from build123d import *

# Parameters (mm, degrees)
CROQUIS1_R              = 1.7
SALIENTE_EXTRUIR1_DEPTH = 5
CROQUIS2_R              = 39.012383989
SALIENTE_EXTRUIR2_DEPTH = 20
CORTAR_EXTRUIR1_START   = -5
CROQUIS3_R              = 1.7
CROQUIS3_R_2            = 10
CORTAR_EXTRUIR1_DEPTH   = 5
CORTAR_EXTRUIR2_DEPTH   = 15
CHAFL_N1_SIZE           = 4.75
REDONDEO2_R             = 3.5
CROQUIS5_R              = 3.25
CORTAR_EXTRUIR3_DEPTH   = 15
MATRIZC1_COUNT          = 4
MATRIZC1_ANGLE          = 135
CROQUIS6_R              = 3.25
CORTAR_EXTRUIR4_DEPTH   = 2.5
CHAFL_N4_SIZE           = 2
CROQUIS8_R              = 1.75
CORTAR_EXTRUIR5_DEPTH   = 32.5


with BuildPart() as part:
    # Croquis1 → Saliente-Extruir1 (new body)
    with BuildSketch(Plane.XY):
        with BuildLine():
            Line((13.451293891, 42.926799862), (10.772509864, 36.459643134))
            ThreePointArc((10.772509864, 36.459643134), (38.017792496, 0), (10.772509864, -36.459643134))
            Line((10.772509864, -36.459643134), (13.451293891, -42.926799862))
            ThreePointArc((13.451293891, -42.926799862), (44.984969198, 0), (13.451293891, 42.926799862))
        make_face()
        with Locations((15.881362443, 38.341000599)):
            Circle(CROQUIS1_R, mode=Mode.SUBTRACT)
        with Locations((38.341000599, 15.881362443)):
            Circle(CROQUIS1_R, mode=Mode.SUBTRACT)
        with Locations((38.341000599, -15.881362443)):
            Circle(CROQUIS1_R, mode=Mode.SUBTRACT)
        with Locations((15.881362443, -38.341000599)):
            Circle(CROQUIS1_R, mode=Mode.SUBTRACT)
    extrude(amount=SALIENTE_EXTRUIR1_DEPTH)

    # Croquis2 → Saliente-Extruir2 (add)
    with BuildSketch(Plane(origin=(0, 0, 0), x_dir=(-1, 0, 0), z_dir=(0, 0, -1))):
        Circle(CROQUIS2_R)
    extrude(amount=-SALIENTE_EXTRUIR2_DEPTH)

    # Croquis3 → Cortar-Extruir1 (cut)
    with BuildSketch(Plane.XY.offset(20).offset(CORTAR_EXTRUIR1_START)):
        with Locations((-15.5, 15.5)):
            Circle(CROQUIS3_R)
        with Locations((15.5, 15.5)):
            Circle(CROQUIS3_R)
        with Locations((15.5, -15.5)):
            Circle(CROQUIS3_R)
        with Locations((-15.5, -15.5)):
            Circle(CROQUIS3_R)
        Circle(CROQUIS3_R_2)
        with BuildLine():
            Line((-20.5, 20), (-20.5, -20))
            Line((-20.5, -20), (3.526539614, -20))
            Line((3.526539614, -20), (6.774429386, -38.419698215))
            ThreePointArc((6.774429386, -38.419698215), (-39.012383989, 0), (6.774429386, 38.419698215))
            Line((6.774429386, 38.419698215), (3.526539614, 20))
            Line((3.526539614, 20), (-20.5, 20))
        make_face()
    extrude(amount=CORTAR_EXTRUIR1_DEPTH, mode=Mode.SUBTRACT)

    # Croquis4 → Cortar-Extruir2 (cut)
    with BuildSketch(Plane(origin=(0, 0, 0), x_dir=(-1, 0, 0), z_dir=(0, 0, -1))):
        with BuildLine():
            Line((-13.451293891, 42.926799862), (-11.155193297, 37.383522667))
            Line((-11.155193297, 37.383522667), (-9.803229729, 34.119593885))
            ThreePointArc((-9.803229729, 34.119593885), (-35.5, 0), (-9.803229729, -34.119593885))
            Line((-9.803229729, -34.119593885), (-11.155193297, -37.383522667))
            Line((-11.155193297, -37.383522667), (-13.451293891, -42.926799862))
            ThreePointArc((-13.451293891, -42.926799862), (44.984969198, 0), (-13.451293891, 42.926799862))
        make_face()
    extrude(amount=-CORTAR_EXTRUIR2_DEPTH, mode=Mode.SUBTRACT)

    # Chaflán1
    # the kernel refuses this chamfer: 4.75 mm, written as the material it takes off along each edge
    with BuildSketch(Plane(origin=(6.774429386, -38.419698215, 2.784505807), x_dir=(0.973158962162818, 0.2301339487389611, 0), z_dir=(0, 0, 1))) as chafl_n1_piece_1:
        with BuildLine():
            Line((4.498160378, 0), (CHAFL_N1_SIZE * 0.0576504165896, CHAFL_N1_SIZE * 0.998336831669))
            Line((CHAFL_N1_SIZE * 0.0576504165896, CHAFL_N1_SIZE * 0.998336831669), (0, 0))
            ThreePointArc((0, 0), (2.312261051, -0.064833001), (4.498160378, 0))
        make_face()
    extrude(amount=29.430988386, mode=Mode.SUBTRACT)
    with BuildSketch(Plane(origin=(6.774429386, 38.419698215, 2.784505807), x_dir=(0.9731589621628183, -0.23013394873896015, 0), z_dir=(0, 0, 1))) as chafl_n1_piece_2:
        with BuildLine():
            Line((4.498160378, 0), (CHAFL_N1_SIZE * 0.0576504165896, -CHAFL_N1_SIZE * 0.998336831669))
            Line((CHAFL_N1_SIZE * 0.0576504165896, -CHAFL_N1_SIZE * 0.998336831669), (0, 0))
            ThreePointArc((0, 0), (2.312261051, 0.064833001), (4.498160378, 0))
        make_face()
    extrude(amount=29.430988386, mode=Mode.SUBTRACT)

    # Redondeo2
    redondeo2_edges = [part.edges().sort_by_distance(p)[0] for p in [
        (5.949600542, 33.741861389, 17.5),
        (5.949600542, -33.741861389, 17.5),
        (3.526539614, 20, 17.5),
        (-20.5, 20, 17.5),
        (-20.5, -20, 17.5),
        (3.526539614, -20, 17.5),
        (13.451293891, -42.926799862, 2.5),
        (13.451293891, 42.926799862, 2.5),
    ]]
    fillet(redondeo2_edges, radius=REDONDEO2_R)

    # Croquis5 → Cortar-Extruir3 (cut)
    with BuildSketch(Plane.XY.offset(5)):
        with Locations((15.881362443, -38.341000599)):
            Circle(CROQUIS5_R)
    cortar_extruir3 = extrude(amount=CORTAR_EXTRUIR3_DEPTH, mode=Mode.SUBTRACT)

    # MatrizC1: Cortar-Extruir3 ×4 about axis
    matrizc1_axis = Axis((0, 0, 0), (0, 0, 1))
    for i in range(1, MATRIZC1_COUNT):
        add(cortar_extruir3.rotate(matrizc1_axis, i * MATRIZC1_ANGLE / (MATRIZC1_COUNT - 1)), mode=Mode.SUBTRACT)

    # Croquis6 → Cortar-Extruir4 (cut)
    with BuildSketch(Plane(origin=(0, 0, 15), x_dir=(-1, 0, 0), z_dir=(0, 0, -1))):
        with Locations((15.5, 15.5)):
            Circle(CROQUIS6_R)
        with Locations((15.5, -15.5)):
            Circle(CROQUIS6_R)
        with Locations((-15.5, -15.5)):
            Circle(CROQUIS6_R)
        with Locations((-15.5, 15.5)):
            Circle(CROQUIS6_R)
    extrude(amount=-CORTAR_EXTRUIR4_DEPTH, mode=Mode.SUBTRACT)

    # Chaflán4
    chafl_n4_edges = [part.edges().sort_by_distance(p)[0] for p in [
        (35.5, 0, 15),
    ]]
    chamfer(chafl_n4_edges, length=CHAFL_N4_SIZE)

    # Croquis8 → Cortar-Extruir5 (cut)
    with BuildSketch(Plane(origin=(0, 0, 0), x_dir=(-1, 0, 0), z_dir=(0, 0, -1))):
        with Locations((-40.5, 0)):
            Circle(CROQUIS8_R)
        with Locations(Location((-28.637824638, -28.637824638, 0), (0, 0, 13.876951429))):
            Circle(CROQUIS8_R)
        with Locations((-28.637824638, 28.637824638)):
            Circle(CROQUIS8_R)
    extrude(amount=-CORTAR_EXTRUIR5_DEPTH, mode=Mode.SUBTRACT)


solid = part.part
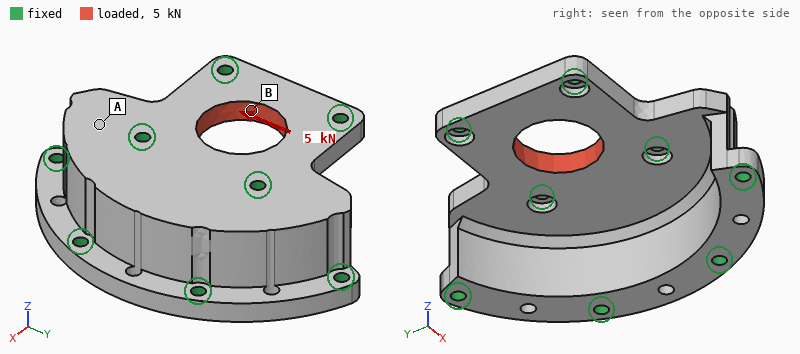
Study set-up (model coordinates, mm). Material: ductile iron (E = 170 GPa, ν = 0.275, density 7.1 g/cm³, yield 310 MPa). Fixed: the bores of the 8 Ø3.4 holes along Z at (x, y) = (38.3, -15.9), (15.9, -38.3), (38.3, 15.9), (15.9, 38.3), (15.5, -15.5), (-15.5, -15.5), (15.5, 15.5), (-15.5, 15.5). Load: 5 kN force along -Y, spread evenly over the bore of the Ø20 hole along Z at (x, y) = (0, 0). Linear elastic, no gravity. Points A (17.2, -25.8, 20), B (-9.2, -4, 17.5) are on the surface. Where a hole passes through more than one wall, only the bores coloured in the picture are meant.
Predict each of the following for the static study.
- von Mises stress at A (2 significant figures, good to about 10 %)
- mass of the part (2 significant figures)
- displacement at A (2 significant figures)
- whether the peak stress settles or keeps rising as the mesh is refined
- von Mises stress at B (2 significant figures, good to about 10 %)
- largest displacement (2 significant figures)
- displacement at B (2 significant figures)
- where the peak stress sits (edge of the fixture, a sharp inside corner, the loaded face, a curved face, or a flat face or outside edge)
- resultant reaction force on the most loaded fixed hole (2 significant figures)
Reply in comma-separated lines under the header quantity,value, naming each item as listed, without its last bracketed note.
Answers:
quantity,value
von Mises stress at A,9.3 MPa
mass of the part,150 g
displacement at A,1.4 µm
whether the peak stress settles or keeps rising as the mesh is refined,keeps rising
von Mises stress at B,31 MPa
largest displacement,4.1 µm
displacement at B,2.6 µm
where the peak stress sits,edge of the fixture
resultant reaction force on the most loaded fixed hole,1.4 kN
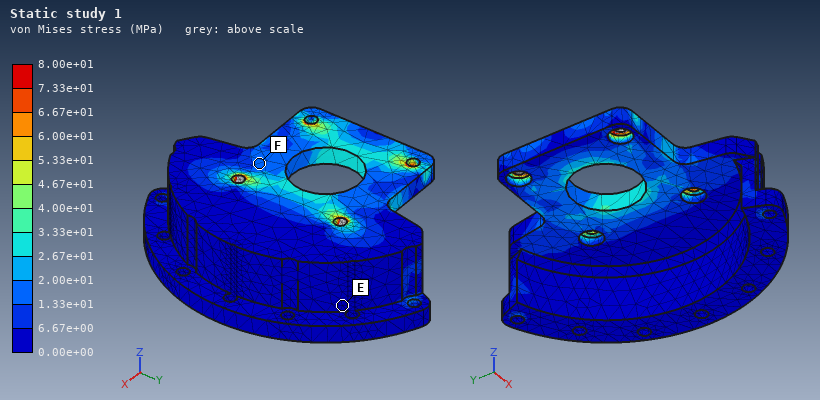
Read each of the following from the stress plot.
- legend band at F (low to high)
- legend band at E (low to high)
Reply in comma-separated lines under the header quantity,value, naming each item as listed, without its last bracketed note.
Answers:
quantity,value
legend band at F,1.33e+01 to 2.00e+01 MPa
legend band at E,0.00e+00 to 6.67e+00 MPa
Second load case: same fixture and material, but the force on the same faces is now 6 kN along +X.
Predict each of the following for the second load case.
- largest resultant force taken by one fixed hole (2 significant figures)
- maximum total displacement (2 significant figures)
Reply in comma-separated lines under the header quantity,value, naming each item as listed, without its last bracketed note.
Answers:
quantity,value
largest resultant force taken by one fixed hole,1.6 kN
maximum total displacement,6.0 µm
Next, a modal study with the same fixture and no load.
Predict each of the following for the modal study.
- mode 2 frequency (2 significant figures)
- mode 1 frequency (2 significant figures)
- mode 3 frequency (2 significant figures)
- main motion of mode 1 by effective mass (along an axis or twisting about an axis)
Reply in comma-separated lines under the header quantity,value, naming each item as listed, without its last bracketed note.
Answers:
quantity,value
mode 2 frequency,20 kHz
mode 1 frequency,17 kHz
mode 3 frequency,20 kHz
main motion of mode 1 by effective mass,along Z
